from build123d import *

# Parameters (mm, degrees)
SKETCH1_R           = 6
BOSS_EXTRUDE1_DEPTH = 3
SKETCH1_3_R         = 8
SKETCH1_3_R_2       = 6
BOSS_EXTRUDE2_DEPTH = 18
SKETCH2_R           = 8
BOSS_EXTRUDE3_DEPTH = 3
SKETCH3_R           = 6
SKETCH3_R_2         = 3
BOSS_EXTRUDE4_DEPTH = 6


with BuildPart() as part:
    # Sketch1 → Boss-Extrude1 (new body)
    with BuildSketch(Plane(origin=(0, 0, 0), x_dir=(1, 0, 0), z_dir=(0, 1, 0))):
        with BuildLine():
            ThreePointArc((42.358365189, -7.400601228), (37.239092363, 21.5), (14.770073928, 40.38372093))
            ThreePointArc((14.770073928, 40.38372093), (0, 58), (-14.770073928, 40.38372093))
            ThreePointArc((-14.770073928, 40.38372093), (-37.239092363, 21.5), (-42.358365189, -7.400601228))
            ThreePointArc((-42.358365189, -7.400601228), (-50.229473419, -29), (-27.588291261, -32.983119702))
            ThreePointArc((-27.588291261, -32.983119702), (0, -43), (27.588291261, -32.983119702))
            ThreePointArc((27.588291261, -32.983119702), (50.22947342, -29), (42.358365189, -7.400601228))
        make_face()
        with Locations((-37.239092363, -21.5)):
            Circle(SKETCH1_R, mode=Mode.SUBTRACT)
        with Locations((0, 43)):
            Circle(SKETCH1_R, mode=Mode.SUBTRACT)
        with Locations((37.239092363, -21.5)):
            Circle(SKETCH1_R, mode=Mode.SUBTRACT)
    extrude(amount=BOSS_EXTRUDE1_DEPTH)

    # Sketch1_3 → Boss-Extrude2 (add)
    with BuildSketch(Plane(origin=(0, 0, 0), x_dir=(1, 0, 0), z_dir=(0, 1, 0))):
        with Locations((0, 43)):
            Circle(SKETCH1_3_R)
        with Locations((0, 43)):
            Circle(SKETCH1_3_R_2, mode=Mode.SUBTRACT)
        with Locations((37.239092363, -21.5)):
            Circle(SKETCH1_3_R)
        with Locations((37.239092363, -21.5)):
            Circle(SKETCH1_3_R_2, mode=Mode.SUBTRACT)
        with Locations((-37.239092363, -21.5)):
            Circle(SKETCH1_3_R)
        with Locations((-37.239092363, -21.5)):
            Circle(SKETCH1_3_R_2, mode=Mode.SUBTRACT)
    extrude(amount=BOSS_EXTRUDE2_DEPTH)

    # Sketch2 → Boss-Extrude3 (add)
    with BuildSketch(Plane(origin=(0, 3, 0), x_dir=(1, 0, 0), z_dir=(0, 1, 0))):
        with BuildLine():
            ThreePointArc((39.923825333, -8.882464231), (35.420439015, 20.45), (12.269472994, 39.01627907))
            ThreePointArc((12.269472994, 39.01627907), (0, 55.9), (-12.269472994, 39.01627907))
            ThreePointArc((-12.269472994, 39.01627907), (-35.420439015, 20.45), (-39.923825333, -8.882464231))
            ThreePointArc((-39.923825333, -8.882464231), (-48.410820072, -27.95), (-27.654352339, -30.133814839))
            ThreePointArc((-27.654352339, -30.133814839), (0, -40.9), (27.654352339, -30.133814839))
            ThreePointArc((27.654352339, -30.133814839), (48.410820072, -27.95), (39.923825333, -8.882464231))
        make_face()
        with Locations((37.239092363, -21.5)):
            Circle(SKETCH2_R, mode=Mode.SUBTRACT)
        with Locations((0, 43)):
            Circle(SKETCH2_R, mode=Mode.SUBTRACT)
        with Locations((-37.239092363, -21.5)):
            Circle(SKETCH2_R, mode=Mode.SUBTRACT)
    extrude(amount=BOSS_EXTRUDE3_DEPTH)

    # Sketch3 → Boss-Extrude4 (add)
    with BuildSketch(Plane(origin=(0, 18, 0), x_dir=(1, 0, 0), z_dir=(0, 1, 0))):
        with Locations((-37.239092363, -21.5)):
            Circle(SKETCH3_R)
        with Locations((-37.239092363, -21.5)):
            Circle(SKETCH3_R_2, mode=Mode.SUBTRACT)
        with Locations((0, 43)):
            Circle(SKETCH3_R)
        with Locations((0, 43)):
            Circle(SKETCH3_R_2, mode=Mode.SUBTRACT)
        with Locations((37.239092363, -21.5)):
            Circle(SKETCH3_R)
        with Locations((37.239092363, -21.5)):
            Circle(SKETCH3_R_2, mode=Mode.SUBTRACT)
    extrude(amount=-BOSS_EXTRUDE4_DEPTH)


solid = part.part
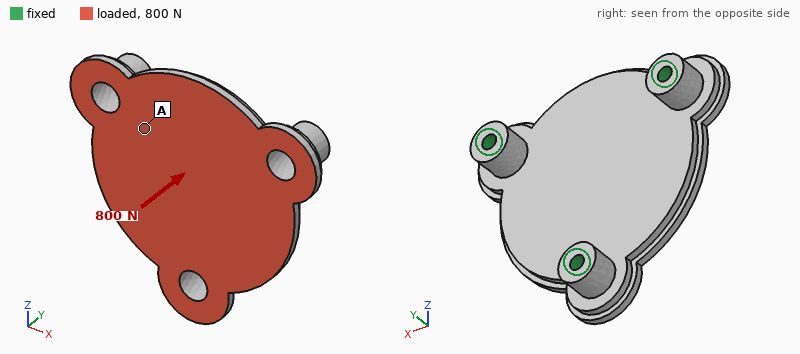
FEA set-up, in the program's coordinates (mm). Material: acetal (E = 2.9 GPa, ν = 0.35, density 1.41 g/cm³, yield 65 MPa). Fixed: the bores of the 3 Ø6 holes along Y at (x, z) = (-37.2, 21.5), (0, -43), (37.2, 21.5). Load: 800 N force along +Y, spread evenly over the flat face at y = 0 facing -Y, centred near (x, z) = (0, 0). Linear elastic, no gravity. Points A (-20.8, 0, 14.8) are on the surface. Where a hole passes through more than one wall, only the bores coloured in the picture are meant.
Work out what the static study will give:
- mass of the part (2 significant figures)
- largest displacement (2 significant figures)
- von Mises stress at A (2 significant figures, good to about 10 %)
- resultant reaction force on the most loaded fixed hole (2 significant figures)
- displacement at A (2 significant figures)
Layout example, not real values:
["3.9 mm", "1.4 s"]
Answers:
["60 g", "0.29 mm", "4.4 MPa", "300 N", "0.15 mm"]
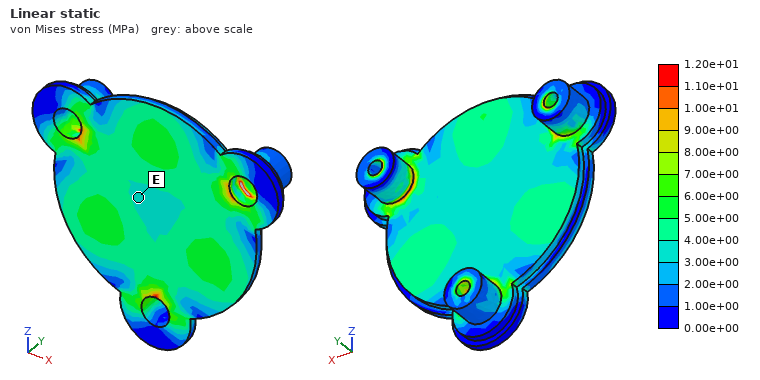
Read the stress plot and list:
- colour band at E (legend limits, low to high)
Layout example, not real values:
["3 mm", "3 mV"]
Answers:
["3.00e+00 to 4.00e+00 MPa"]
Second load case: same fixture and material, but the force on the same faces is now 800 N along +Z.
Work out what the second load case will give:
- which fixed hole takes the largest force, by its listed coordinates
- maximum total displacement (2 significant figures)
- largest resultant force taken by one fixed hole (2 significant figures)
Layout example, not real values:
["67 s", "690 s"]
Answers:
["(0, -43)", "0.20 mm", "310 N"]
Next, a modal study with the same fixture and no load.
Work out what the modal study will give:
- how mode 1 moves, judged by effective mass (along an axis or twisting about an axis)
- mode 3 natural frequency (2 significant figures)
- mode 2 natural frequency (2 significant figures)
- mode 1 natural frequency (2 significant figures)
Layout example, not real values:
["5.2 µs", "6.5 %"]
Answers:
["along Y", "1400 Hz", "1400 Hz", "1300 Hz"]
